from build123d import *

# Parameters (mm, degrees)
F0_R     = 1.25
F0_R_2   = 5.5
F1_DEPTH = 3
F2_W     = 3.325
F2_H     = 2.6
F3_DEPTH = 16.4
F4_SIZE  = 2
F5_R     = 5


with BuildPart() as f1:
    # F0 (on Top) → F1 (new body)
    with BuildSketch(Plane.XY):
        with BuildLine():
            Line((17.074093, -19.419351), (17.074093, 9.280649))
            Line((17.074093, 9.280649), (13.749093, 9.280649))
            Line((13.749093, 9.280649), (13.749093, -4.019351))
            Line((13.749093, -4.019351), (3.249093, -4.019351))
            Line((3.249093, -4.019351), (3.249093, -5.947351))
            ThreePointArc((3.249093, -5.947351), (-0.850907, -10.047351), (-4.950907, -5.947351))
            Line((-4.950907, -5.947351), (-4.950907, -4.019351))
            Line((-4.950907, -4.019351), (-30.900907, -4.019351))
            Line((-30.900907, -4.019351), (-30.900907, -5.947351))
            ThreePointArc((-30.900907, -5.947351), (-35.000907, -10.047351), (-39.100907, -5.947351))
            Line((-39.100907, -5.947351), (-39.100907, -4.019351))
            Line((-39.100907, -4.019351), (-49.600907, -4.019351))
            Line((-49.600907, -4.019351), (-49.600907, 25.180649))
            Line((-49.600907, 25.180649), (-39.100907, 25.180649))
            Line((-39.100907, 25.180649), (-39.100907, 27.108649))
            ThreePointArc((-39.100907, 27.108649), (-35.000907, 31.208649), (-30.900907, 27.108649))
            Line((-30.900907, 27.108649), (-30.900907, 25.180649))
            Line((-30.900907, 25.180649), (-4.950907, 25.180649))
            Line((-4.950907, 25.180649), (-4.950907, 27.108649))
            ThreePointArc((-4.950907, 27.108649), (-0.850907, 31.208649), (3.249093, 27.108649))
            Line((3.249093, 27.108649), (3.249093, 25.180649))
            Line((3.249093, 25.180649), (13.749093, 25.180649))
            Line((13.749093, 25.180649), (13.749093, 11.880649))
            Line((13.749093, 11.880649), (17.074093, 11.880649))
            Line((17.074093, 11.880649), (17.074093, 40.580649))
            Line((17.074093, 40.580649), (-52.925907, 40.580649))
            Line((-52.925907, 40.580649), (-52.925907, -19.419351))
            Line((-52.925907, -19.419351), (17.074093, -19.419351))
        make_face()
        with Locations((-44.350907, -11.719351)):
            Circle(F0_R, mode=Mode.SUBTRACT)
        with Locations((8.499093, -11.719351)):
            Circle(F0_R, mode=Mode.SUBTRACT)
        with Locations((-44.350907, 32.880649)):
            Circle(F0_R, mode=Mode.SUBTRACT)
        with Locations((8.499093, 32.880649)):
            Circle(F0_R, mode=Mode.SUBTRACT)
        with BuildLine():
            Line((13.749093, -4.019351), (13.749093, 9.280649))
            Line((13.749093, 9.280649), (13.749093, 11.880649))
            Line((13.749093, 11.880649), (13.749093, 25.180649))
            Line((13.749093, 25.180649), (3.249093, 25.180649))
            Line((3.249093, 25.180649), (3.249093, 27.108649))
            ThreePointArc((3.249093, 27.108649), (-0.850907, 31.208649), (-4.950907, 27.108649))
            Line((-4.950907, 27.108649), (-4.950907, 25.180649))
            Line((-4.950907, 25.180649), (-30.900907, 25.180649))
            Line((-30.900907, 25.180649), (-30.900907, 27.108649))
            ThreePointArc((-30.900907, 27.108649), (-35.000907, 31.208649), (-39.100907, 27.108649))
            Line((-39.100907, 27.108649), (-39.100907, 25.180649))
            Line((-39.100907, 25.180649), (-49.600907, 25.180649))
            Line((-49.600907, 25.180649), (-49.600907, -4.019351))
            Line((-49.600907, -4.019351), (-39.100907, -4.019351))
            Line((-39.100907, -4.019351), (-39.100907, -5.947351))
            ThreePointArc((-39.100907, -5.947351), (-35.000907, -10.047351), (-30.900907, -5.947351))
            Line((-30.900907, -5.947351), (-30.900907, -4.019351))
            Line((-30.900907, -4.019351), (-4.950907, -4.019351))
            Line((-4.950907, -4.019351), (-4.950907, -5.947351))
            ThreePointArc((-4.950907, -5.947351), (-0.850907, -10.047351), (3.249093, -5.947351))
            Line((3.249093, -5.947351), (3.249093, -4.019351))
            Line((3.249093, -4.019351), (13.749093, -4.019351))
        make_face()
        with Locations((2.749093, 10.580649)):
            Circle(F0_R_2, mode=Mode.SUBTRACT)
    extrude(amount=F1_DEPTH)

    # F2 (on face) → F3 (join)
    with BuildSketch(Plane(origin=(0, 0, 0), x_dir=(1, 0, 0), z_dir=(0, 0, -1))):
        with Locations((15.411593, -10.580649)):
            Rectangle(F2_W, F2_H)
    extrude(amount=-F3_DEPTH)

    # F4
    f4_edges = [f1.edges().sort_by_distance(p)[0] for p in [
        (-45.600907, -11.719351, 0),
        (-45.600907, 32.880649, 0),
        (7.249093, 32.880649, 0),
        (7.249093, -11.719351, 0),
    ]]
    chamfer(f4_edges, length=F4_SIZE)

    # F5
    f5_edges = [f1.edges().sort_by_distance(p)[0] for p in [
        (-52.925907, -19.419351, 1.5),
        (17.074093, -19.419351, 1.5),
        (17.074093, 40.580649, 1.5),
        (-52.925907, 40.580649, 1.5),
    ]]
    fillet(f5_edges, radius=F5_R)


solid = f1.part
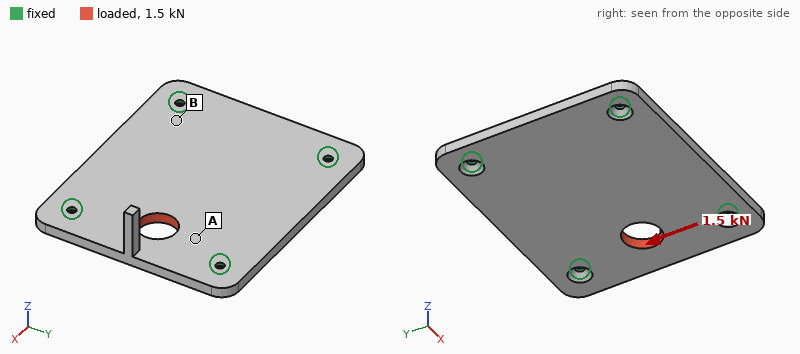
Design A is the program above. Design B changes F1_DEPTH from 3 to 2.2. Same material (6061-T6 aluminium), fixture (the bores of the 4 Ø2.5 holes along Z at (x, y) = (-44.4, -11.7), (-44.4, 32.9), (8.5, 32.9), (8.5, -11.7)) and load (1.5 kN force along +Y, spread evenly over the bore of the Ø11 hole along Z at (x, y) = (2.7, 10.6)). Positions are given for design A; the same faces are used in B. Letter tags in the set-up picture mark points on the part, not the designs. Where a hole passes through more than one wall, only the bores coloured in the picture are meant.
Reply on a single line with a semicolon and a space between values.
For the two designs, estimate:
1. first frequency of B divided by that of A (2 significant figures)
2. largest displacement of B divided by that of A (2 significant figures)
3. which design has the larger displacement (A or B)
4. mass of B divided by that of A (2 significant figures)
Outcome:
0.73; 3.1; B; 0.73
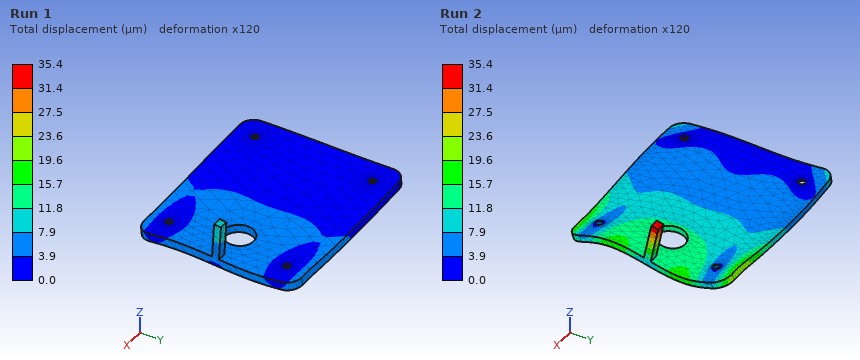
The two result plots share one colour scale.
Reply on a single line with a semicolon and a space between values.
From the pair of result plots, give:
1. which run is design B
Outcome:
Run 2
